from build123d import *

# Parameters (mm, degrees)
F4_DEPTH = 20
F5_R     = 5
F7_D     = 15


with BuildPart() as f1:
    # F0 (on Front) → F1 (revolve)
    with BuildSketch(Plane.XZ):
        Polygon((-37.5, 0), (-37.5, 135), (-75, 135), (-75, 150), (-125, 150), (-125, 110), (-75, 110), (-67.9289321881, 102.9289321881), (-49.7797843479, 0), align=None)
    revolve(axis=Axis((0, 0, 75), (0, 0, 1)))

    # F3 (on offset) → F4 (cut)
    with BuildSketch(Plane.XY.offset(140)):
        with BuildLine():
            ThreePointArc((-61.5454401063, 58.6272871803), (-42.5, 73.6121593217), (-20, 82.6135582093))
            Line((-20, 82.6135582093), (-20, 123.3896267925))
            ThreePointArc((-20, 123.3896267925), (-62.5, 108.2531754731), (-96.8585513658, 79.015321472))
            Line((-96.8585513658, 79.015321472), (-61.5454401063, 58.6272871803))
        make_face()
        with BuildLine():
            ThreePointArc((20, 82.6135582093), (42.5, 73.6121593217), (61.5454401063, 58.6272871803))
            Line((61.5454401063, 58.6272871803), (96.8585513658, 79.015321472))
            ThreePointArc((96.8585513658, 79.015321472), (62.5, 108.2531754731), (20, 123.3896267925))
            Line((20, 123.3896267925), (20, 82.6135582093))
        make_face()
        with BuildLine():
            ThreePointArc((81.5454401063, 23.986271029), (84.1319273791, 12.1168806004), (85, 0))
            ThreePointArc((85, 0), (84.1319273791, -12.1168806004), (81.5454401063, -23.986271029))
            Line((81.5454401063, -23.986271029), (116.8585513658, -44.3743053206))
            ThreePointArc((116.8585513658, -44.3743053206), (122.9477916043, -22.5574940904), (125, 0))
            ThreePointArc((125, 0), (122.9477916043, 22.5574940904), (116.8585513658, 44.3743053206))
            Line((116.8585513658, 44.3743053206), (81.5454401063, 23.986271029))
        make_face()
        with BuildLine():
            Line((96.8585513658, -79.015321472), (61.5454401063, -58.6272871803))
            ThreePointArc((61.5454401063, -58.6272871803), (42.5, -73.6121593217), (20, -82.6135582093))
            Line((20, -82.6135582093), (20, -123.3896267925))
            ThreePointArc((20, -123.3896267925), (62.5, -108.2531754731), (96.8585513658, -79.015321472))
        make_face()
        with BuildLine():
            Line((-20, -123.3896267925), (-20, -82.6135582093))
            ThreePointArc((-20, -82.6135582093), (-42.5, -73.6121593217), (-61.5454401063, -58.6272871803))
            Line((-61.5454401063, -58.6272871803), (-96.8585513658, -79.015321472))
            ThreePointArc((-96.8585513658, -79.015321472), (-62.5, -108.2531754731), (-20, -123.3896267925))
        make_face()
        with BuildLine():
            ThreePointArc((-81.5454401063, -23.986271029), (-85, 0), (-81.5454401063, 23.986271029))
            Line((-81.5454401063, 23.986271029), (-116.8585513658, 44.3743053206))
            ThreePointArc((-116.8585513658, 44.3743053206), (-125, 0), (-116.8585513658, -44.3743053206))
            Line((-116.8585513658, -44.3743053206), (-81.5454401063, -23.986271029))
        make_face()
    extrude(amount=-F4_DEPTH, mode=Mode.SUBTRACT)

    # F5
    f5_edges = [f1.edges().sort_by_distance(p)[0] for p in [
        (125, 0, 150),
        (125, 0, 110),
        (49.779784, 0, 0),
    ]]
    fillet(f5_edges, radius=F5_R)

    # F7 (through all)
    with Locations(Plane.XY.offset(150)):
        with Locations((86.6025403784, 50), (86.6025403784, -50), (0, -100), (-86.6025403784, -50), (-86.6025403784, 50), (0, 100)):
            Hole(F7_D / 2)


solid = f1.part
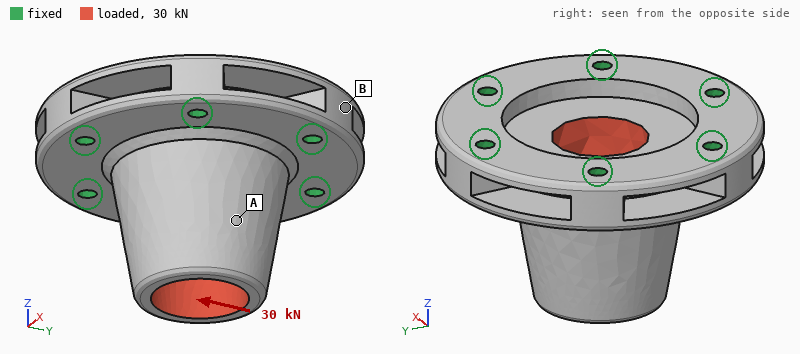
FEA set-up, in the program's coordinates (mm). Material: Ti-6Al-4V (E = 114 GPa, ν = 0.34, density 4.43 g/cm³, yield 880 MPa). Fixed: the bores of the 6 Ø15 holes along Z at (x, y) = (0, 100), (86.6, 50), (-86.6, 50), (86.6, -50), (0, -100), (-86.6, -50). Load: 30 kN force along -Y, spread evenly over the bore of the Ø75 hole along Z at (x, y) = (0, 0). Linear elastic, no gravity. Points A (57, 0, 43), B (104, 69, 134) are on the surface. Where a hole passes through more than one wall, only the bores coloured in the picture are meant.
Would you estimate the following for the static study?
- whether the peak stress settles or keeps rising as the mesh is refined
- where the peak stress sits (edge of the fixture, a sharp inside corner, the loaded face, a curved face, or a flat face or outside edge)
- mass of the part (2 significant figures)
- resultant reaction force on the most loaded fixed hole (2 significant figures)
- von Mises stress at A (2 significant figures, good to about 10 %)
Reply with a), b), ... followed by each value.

a) keeps rising
b) edge of the fixture
c) 8.7 kg
d) 10 kN
e) 4.1 MPa
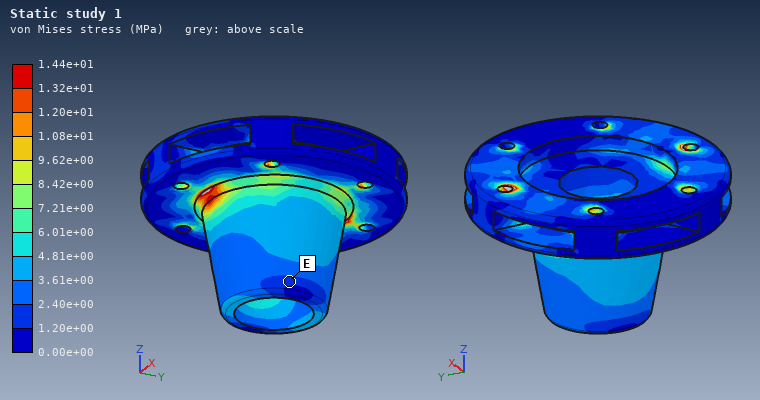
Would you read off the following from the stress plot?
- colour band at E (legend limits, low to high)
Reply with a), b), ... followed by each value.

a) 1.20e+00 to 2.40e+00 MPa
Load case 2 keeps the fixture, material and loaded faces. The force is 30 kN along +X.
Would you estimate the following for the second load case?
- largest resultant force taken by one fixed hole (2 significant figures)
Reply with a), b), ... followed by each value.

a) 9.0 kN
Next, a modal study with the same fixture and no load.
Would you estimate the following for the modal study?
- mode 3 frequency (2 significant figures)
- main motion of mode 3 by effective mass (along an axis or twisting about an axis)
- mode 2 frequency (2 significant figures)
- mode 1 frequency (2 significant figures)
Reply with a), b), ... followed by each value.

a) 5700 Hz
b) along Z
c) 4300 Hz
d) 4300 Hz
